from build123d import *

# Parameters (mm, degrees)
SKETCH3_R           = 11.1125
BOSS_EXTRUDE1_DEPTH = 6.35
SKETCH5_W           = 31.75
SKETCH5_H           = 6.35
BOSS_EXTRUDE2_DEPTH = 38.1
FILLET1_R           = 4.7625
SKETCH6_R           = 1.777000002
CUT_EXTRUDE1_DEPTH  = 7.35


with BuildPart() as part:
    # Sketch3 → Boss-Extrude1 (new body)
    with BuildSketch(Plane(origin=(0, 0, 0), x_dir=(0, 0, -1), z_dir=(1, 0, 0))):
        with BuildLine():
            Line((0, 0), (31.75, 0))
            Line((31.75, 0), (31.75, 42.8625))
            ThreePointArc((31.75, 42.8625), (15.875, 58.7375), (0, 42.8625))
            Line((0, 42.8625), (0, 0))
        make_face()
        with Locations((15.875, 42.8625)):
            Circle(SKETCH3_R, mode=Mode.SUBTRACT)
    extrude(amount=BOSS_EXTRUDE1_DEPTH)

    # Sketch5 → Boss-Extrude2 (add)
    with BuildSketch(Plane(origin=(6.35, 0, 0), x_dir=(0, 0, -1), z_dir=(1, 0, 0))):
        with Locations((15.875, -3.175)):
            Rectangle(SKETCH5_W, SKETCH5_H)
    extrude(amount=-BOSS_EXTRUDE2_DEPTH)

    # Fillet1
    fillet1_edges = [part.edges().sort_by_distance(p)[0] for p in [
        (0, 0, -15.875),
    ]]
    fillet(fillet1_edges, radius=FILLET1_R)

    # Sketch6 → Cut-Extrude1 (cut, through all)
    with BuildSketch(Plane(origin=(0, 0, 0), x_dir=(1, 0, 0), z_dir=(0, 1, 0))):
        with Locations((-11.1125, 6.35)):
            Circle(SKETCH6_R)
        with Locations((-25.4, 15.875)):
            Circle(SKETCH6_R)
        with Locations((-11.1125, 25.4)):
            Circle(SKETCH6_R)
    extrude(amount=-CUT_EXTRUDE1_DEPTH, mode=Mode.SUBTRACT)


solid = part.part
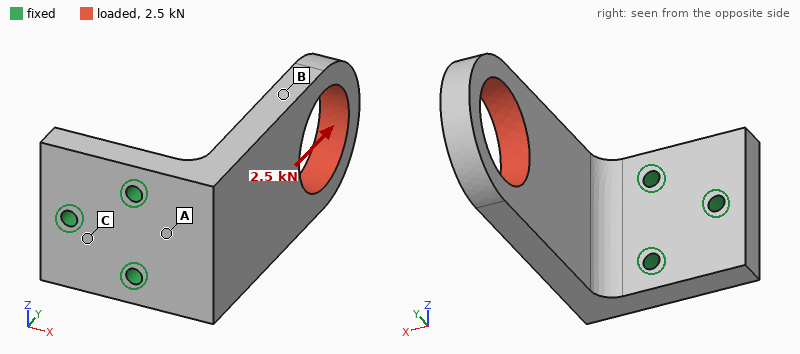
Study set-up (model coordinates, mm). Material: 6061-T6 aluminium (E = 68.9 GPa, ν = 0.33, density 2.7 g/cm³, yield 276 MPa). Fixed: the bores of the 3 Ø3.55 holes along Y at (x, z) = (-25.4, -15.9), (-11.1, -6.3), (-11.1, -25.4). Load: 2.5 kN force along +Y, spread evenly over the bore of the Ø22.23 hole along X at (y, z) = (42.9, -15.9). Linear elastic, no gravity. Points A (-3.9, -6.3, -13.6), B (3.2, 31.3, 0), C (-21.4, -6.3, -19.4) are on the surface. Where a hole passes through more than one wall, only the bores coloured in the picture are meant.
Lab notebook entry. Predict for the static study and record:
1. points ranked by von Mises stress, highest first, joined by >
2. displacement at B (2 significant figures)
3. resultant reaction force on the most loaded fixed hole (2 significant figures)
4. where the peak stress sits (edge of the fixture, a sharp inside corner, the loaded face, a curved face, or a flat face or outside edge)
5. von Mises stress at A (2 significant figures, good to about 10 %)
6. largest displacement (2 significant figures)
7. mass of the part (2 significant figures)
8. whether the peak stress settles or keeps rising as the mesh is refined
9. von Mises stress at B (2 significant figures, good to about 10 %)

A > B > C
0.20 mm
1.5 kN
edge of the fixture
65 MPa
0.35 mm
44 g
keeps rising
35 MPa
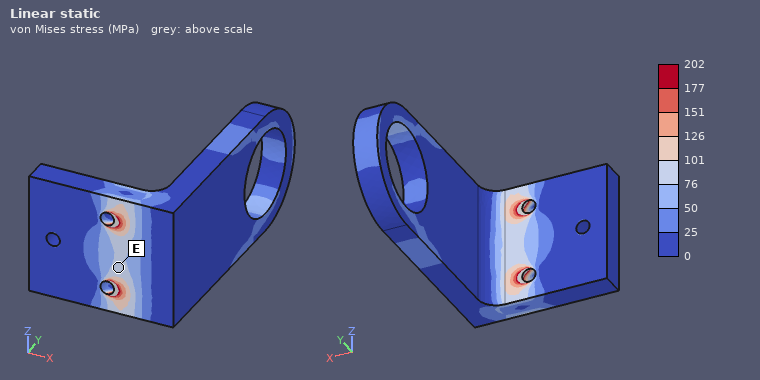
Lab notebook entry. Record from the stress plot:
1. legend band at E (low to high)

76 to 101 MPa
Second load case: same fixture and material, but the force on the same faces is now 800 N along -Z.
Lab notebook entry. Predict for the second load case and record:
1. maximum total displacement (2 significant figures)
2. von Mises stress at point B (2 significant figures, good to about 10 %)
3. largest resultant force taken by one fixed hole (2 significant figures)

0.24 mm
33 MPa
1.8 kN
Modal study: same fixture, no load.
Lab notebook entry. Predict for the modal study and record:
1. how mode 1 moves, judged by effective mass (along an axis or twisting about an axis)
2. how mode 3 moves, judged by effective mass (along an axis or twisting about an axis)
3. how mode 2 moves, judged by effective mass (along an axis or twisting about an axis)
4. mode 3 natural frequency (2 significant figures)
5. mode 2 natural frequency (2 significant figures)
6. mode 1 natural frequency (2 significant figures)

along X
along Y
along Z
5800 Hz
3300 Hz
1500 Hz
